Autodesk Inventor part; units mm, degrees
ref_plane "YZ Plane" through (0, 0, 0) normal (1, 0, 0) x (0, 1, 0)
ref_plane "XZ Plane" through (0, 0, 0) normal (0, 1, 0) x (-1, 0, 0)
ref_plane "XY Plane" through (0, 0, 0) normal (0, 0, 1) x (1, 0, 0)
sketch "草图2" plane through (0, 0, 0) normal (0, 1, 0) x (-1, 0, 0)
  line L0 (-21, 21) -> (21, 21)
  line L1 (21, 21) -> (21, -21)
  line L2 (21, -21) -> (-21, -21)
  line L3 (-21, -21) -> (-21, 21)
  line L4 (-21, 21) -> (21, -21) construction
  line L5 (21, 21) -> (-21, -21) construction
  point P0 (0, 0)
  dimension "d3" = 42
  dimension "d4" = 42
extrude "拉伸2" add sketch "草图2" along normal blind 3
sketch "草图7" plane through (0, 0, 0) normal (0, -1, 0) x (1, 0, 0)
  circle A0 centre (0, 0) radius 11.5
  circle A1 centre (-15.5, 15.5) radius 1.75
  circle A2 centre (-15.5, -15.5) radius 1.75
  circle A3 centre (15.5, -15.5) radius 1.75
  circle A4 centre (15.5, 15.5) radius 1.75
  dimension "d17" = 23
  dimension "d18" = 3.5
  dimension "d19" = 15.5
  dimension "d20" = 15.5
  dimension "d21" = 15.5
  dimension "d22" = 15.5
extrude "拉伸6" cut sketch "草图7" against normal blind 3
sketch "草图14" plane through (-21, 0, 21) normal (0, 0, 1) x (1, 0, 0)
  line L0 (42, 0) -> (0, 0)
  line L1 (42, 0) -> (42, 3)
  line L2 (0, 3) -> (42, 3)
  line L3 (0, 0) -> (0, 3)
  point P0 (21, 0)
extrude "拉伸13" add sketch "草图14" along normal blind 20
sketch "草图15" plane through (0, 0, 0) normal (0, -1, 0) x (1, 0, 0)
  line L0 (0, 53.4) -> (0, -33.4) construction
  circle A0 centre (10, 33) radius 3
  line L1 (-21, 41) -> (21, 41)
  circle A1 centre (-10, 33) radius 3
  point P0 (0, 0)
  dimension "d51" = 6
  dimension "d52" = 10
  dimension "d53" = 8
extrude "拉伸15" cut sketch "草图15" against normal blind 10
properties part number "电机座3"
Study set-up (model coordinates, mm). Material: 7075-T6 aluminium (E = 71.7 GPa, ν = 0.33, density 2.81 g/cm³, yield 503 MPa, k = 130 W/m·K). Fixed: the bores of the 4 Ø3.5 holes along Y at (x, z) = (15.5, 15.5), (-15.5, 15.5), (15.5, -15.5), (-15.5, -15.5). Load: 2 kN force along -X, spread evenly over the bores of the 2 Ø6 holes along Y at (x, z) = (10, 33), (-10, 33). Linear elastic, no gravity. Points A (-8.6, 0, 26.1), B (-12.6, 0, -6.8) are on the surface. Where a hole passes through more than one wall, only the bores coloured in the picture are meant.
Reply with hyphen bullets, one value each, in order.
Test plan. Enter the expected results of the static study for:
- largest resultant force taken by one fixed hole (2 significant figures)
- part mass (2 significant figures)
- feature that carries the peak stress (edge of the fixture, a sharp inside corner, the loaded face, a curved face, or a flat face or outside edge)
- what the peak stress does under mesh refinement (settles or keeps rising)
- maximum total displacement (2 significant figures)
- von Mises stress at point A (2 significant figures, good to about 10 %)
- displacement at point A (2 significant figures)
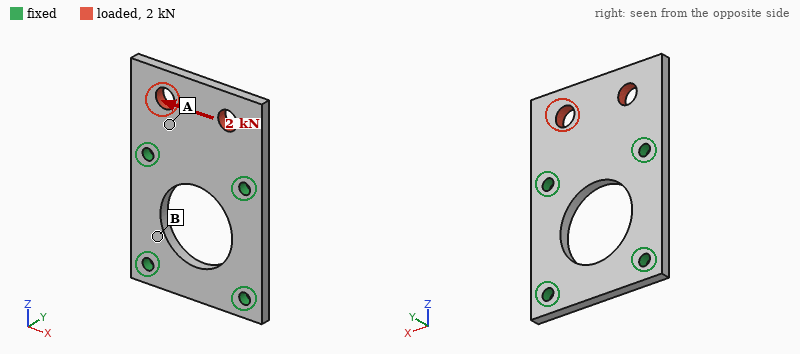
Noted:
- 1.4 kN
- 18 g
- edge of the fixture
- keeps rising
- 23 µm
- 44 MPa
- 9.8 µm
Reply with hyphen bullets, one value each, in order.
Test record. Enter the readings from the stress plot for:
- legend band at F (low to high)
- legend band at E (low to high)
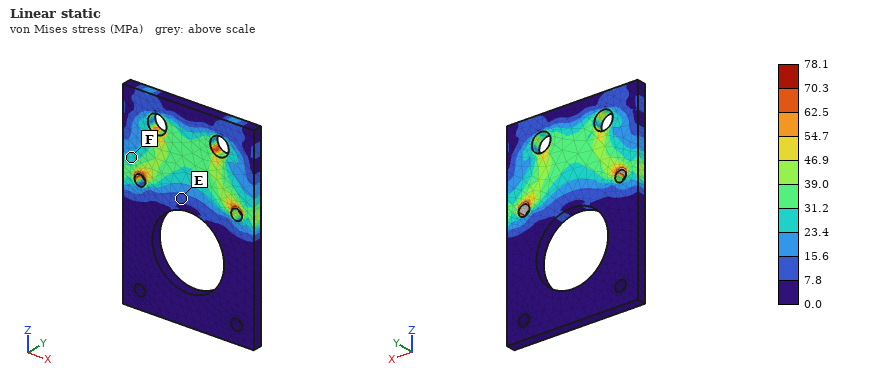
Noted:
- 23.4 to 31.2 MPa
- 7.8 to 15.6 MPa
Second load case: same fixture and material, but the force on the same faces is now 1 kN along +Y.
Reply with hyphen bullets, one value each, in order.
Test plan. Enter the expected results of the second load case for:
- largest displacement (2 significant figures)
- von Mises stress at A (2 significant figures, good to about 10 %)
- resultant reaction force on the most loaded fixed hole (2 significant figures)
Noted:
- 0.57 mm
- 110 MPa
- 540 N
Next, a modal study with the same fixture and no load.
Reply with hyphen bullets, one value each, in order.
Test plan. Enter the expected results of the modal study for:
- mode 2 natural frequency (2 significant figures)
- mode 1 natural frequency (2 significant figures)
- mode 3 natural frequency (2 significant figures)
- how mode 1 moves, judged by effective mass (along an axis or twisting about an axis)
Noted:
- 6500 Hz
- 3600 Hz
- 12 kHz
- along Y
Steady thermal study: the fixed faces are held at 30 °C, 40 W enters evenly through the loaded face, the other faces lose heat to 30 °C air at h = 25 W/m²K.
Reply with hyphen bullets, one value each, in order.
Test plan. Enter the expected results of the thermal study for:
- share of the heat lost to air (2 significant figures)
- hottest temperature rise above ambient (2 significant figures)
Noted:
- 5.5 %
- 58 K
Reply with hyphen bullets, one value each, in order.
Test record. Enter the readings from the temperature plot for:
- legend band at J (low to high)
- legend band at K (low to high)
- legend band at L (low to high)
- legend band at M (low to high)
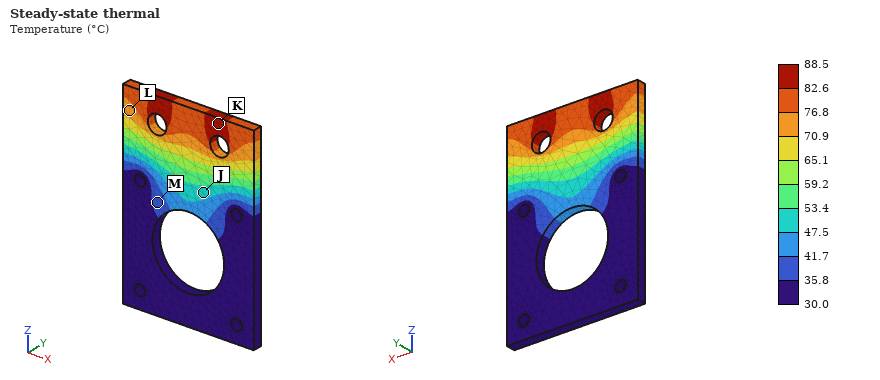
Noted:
- 47.5 to 53.4 °C
- 82.6 to 88.5 °C
- 70.9 to 76.8 °C
- 35.8 to 41.7 °C
